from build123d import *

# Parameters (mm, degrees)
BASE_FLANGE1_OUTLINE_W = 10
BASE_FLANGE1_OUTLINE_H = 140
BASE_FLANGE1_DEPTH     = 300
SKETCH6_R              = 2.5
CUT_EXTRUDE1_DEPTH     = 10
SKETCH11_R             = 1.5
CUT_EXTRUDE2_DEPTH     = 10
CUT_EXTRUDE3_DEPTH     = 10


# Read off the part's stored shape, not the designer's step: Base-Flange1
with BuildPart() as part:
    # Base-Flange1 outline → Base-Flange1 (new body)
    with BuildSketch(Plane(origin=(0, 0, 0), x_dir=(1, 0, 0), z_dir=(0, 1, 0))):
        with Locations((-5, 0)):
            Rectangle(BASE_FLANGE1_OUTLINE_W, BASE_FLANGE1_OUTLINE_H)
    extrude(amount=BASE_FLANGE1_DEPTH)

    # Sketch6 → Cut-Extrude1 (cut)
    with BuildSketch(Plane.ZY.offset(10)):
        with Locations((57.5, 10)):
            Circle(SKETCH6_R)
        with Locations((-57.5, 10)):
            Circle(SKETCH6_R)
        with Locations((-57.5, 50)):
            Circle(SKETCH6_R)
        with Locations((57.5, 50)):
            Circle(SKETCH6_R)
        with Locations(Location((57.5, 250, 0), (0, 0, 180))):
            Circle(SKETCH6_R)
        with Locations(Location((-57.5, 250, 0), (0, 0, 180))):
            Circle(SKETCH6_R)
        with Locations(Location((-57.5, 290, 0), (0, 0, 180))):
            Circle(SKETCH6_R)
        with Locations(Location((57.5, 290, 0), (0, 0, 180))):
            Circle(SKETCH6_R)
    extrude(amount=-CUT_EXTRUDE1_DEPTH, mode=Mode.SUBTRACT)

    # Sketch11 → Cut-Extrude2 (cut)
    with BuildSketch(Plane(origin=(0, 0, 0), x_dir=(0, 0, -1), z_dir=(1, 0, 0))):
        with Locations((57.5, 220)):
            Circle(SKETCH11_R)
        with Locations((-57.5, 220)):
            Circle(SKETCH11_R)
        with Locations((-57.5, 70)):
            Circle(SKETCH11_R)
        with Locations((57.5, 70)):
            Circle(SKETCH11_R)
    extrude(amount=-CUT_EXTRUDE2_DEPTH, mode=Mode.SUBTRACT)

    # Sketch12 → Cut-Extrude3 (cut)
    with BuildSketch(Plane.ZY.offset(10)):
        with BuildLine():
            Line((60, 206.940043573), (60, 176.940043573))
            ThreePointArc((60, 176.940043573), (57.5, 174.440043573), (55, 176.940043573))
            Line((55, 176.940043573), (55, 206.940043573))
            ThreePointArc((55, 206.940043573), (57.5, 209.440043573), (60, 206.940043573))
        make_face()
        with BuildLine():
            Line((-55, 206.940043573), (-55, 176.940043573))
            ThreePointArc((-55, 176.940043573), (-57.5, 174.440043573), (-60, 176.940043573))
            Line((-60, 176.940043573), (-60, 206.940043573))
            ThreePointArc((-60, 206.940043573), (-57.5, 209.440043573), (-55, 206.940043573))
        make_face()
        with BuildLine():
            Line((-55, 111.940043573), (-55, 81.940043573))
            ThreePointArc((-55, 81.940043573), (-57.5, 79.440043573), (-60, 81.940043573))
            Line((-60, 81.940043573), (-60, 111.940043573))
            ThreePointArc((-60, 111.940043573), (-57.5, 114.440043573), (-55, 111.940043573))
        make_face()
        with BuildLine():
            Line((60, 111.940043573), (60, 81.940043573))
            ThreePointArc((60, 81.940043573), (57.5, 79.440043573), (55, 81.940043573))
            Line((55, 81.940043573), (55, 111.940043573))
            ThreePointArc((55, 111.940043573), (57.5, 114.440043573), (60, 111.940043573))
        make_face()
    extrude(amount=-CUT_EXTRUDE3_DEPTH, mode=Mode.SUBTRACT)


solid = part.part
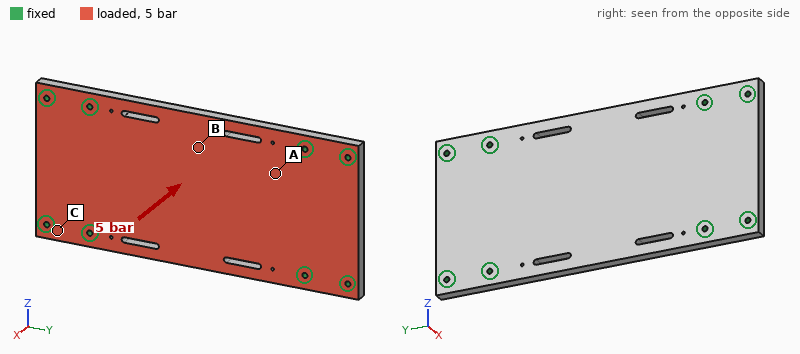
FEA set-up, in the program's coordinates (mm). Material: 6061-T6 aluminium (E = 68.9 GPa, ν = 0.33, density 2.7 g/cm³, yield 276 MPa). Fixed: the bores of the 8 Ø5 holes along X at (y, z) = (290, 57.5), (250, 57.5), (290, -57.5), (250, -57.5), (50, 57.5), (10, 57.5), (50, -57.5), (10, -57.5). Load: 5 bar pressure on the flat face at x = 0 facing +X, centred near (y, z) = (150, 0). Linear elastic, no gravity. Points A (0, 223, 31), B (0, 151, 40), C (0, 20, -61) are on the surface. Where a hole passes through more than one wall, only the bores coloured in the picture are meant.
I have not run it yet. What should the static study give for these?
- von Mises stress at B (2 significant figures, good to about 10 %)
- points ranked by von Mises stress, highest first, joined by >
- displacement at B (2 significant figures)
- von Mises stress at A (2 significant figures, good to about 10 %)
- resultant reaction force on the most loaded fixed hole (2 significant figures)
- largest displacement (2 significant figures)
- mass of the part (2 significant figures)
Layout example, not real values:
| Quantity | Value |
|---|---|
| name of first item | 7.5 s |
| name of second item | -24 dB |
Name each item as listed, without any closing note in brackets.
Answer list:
| Quantity | Value |
|---|---|
| von Mises stress at B | 52 MPa |
| points ranked by von Mises stress, highest first, joined by > | B > A > C |
| displacement at B | 0.51 mm |
| von Mises stress at A | 27 MPa |
| resultant reaction force on the most loaded fixed hole | 5.3 kN |
| largest displacement | 0.52 mm |
| mass of the part | 1.1 kg |
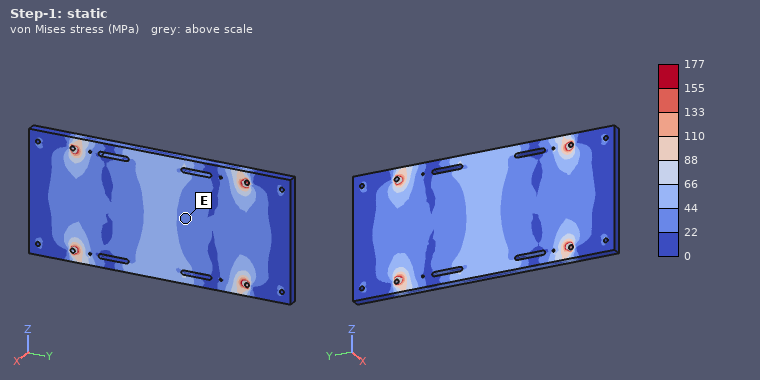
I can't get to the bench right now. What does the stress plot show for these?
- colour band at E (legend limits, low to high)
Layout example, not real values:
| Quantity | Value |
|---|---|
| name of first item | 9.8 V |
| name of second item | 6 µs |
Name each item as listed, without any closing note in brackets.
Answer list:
| Quantity | Value |
|---|---|
| colour band at E | 22 to 44 MPa |
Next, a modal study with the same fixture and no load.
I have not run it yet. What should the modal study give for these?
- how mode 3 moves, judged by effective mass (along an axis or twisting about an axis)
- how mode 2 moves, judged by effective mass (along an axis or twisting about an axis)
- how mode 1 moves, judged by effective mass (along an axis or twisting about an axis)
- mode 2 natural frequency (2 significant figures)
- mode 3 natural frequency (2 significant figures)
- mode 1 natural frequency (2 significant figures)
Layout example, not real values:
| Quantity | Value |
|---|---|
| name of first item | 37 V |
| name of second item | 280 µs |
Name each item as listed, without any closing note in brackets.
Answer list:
| Quantity | Value |
|---|---|
| how mode 3 moves, judged by effective mass | twisting about Z |
| how mode 2 moves, judged by effective mass | twisting about Y |
| how mode 1 moves, judged by effective mass | along X |
| mode 2 natural frequency | 1700 Hz |
| mode 3 natural frequency | 2700 Hz |
| mode 1 natural frequency | 1100 Hz |
